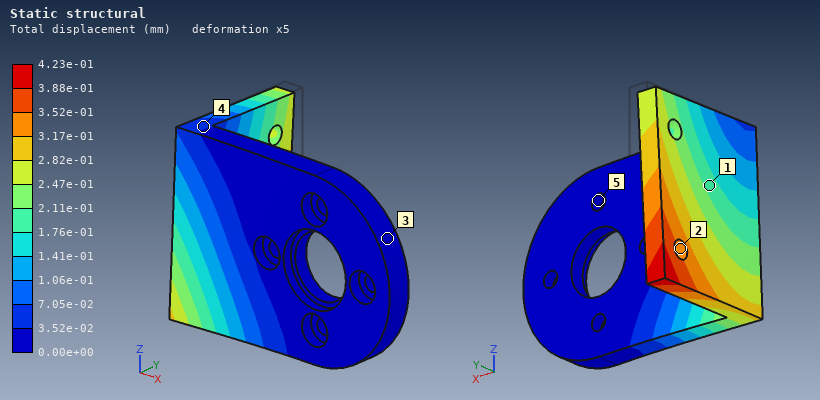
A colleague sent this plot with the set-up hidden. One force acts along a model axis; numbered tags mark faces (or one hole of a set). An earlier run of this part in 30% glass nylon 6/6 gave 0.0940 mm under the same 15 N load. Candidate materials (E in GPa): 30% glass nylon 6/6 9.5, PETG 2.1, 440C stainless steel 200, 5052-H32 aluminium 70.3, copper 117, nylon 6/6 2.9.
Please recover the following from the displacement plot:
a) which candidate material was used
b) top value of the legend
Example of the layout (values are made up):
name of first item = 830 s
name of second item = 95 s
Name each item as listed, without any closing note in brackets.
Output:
which candidate material was used = PETG
top value of the legend = 4.23e-01 mm
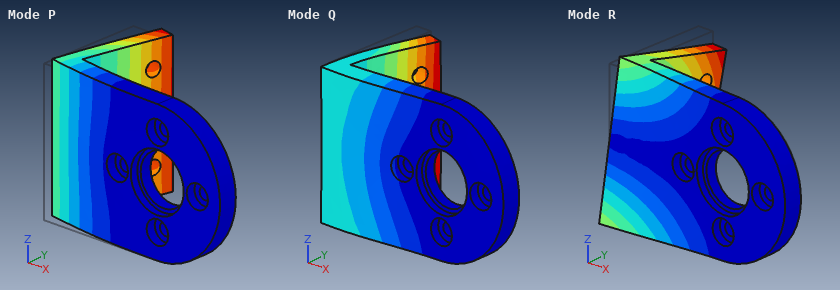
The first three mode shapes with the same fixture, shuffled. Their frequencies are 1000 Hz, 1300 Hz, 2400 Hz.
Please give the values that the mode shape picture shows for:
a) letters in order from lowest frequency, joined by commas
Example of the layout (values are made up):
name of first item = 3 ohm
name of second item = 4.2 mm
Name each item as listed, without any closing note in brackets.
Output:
letters in order from lowest frequency, joined by commas = P, R, Q
